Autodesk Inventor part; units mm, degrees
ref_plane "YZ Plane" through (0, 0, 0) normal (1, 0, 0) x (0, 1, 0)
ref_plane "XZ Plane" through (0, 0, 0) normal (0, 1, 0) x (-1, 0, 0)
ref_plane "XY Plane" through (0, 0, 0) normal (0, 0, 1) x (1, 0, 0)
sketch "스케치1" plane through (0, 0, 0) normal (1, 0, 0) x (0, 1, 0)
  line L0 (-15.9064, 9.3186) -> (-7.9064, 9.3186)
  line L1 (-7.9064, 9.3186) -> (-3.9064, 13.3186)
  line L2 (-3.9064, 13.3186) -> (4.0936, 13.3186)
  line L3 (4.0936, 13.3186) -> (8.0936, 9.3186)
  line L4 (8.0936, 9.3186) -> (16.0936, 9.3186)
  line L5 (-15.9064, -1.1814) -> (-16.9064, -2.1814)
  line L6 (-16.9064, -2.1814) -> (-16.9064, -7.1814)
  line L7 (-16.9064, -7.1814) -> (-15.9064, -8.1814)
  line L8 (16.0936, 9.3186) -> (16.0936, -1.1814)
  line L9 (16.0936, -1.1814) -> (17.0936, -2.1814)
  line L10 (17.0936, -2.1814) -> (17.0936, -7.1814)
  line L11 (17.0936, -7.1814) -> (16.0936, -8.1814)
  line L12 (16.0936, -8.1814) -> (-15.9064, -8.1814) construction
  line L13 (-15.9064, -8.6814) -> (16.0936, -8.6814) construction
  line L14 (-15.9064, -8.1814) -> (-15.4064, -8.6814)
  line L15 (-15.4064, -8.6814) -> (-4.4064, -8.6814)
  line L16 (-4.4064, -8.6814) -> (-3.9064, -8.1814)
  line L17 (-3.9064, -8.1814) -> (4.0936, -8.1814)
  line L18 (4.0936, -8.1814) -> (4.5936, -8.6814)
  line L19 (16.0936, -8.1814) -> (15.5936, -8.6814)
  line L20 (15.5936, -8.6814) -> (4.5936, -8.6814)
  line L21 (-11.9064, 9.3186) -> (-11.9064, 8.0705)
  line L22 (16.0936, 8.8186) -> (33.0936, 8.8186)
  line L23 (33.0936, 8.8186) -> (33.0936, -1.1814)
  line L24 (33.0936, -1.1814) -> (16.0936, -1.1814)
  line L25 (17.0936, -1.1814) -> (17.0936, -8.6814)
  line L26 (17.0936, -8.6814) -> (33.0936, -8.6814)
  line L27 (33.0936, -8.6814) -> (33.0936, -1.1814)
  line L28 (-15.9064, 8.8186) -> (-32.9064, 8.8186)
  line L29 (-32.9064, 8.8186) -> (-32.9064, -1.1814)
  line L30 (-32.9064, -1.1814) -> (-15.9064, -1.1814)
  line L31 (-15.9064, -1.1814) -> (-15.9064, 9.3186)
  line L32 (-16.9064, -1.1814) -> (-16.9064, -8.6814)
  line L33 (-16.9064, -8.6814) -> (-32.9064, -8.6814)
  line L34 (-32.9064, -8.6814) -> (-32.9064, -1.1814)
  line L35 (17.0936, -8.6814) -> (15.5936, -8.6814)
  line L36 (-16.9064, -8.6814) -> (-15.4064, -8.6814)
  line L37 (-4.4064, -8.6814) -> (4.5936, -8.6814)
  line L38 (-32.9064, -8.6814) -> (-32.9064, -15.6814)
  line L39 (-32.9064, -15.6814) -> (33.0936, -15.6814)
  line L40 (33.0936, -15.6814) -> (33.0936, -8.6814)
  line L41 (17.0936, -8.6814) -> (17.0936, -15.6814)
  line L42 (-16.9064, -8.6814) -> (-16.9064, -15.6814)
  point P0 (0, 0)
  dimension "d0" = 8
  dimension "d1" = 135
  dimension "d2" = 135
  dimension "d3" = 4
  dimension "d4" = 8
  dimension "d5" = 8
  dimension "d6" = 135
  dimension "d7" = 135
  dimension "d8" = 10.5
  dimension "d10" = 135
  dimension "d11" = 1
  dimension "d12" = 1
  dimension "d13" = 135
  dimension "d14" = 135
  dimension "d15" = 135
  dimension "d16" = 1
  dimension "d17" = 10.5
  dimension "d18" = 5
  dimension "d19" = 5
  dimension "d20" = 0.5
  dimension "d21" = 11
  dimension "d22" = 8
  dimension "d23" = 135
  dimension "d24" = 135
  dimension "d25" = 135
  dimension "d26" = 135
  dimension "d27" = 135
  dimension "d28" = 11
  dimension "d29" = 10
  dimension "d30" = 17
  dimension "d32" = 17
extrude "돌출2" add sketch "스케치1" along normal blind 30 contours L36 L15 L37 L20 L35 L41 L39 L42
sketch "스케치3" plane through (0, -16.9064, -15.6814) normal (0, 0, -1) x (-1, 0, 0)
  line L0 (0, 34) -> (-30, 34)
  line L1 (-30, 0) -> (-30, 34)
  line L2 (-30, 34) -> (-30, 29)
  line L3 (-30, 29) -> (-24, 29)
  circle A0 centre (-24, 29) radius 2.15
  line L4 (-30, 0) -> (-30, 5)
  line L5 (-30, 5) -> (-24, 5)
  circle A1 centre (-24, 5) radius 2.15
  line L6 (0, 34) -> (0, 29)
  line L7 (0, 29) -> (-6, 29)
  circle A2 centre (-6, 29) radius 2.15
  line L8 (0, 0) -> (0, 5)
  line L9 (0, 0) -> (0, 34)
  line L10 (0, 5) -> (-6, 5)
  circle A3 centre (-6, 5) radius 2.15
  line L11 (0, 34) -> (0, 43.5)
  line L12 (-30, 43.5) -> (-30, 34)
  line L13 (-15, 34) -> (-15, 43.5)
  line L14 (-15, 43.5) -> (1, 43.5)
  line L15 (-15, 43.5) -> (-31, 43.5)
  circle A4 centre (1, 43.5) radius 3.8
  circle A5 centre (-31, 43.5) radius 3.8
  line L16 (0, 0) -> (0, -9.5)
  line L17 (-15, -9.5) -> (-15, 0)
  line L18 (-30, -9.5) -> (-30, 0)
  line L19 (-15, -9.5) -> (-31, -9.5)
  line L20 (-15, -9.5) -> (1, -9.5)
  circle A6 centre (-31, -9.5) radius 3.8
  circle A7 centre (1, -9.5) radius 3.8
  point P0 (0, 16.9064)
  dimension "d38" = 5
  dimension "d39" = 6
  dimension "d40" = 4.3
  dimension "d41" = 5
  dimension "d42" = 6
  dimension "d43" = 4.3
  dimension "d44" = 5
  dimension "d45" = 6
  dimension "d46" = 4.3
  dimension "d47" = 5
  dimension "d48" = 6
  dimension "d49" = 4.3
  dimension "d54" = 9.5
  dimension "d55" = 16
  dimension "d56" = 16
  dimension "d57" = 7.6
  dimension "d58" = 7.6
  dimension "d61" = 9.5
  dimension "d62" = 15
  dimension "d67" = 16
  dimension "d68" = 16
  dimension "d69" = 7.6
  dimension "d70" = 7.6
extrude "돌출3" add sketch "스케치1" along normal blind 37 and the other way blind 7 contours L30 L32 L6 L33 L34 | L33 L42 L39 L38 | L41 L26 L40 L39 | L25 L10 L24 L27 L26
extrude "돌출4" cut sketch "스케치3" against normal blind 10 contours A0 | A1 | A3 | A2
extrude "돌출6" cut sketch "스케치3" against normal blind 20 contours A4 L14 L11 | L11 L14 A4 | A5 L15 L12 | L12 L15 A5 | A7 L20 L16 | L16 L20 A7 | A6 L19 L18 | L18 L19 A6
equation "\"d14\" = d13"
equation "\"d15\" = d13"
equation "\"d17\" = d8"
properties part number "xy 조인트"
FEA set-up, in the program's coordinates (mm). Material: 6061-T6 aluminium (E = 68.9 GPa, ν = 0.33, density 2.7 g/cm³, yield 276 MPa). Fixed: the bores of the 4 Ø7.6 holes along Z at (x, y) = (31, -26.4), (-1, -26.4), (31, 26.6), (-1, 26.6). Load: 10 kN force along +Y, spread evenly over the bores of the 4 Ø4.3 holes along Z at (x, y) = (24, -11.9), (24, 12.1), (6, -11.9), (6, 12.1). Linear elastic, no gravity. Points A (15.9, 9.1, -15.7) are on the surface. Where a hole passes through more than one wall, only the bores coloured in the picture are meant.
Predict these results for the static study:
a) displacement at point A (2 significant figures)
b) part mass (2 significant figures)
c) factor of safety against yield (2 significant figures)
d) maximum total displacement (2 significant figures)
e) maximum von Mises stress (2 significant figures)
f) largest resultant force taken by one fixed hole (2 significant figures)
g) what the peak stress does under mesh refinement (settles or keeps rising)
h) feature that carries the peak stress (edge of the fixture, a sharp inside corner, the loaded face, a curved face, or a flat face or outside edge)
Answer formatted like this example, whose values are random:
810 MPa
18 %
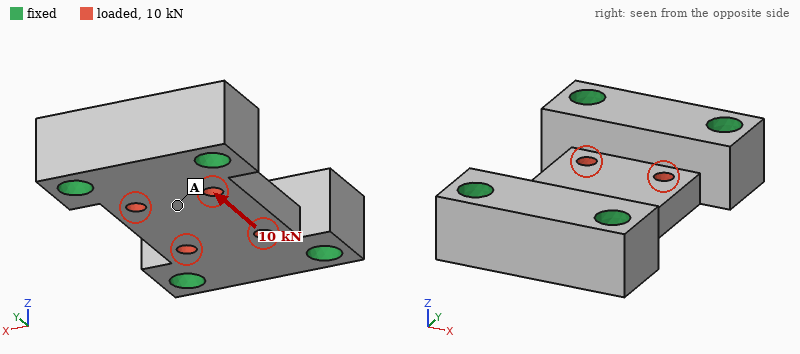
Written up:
5.0 µm
66 g
3.9
7.9 µm
71 MPa
2.6 kN
settles
the loaded face
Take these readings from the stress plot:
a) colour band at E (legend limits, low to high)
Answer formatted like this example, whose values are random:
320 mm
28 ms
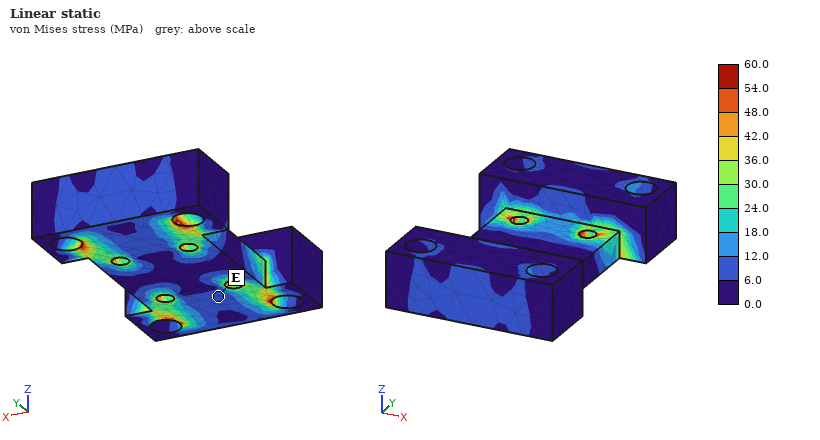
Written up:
6.0 to 12.0 MPa
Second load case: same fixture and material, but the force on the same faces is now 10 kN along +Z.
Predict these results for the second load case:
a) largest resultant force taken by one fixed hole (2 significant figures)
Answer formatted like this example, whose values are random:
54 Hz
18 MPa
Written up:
2.6 kN
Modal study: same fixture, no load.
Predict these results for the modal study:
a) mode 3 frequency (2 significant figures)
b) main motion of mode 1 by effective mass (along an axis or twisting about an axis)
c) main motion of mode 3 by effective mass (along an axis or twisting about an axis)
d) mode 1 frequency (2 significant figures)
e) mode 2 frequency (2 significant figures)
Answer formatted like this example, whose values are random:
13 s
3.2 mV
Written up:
30 kHz
along Z
along X
17 kHz
23 kHz
